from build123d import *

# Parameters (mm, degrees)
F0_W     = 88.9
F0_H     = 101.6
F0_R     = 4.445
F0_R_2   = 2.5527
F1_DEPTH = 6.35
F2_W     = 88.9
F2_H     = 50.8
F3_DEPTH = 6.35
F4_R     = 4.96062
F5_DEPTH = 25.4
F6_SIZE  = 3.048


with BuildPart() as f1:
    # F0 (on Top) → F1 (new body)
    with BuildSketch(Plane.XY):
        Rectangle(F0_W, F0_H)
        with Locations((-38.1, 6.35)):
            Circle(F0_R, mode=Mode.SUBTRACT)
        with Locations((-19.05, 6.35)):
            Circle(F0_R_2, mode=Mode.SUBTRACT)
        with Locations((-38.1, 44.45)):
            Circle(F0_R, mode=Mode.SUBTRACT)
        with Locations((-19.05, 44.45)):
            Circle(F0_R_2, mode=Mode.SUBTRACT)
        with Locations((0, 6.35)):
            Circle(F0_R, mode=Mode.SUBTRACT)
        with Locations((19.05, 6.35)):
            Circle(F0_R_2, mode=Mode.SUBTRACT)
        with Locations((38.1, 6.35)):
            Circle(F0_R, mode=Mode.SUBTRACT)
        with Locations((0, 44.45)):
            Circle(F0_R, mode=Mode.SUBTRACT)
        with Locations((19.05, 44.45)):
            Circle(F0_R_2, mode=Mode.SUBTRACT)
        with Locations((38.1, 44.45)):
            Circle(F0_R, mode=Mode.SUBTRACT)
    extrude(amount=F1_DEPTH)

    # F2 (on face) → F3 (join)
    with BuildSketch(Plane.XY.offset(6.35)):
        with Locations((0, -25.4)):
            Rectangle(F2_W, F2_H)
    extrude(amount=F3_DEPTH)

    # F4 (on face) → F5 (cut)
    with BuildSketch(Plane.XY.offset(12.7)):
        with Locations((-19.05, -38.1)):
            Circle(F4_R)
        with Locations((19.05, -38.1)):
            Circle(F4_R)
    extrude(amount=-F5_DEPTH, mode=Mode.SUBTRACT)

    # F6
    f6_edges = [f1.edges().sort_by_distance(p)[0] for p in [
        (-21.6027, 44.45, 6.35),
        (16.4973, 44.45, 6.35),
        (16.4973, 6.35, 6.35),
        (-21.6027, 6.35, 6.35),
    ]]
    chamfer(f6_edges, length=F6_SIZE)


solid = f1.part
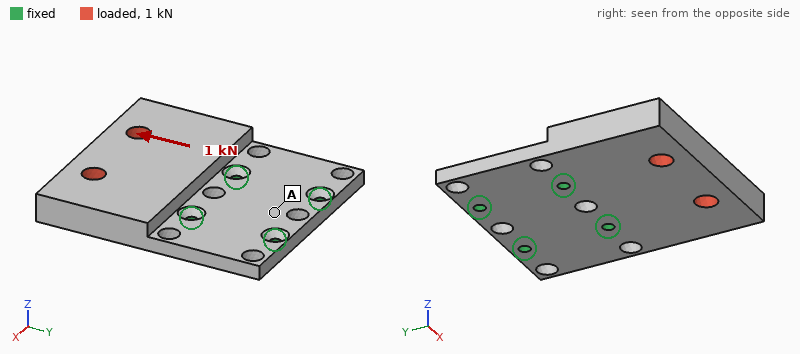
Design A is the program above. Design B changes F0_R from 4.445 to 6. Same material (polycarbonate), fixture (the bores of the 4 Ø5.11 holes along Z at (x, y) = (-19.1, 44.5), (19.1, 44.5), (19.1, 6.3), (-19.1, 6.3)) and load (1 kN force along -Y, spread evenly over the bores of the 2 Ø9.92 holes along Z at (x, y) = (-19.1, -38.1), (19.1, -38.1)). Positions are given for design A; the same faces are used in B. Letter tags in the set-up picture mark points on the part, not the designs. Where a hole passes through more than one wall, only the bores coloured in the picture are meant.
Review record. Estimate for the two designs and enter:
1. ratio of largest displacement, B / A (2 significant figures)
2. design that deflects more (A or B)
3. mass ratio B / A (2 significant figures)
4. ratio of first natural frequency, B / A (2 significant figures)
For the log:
1.1
B
0.98
0.94
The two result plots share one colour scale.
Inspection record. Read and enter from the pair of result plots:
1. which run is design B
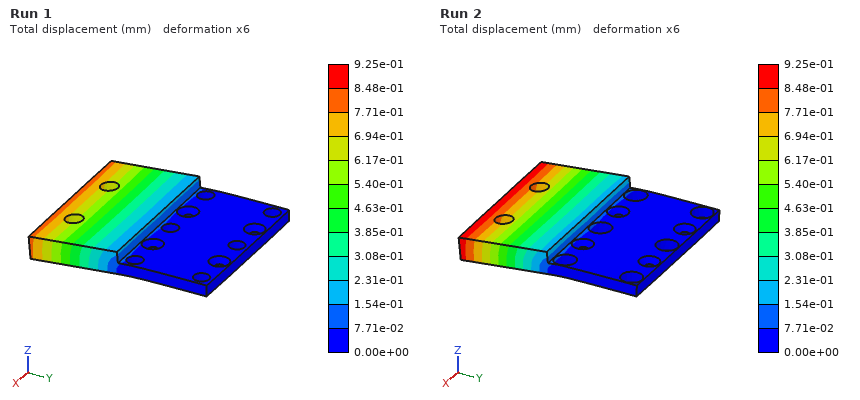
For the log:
Run 2
